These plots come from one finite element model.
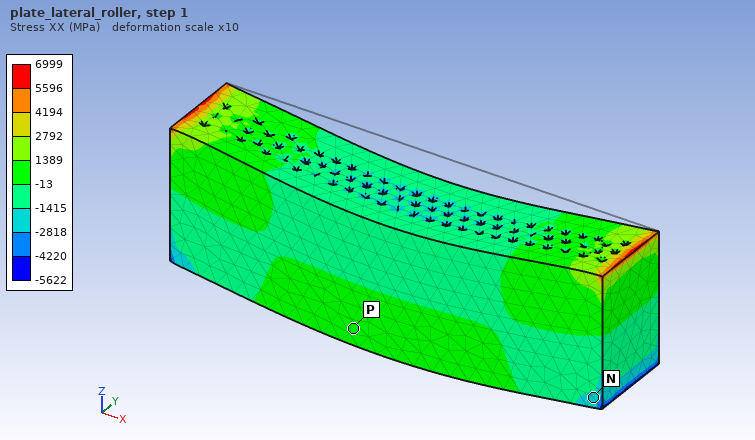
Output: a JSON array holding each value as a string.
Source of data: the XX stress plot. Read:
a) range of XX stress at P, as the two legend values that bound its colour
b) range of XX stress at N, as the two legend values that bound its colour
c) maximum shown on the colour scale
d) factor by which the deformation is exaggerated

["-13 to 1389 MPa", "-2818 to -1415 MPa", "6999 MPa", "10"]
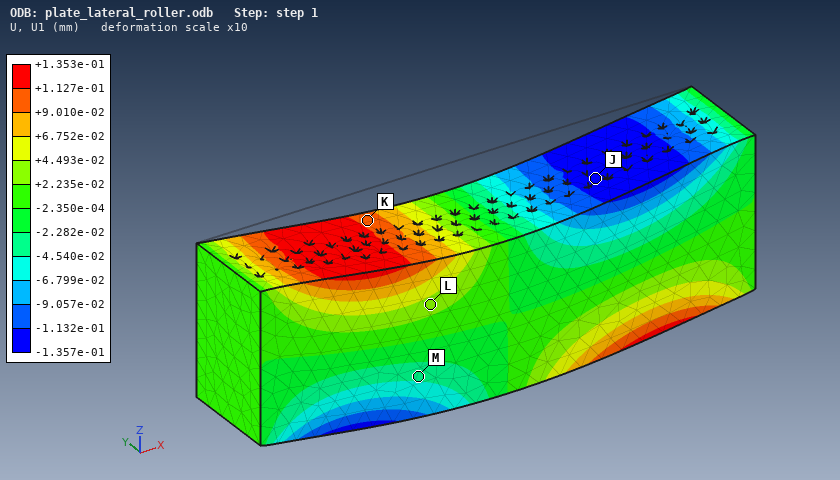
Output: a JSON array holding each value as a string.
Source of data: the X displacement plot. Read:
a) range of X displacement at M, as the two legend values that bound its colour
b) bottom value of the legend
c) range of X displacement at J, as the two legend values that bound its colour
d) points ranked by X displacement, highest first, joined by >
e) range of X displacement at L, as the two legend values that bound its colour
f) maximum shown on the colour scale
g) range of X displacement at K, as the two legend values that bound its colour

["-4.540e-02 to -2.282e-02 mm", "-1.357e-01 mm", "-1.357e-01 to -1.132e-01 mm", "K > L > M > J", "+2.235e-02 to +4.493e-02 mm", "+1.353e-01 mm", "+9.010e-02 to +1.127e-01 mm"]
